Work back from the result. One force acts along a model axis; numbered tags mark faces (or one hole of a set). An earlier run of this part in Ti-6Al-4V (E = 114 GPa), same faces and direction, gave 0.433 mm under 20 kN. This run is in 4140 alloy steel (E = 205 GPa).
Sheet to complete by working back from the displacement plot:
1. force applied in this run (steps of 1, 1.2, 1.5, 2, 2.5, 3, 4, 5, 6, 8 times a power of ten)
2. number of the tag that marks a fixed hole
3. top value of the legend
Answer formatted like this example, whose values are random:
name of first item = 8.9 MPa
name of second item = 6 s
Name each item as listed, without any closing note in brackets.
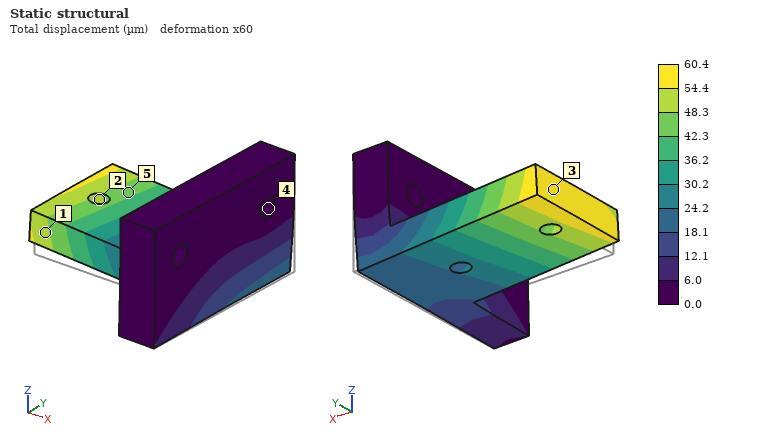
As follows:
force applied in this run = 5 kN
number of the tag that marks a fixed hole = 4
top value of the legend = 60.4 µm
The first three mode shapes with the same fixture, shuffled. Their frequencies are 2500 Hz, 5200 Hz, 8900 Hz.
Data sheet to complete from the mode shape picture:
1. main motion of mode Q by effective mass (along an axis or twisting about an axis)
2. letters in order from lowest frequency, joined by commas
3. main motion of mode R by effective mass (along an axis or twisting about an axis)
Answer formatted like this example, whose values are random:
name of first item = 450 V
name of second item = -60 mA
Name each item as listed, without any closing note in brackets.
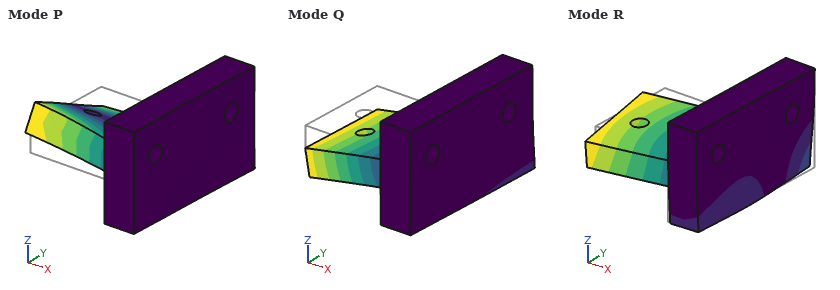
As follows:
main motion of mode Q by effective mass = along Z
letters in order from lowest frequency, joined by commas = Q, R, P
main motion of mode R by effective mass = along Y
